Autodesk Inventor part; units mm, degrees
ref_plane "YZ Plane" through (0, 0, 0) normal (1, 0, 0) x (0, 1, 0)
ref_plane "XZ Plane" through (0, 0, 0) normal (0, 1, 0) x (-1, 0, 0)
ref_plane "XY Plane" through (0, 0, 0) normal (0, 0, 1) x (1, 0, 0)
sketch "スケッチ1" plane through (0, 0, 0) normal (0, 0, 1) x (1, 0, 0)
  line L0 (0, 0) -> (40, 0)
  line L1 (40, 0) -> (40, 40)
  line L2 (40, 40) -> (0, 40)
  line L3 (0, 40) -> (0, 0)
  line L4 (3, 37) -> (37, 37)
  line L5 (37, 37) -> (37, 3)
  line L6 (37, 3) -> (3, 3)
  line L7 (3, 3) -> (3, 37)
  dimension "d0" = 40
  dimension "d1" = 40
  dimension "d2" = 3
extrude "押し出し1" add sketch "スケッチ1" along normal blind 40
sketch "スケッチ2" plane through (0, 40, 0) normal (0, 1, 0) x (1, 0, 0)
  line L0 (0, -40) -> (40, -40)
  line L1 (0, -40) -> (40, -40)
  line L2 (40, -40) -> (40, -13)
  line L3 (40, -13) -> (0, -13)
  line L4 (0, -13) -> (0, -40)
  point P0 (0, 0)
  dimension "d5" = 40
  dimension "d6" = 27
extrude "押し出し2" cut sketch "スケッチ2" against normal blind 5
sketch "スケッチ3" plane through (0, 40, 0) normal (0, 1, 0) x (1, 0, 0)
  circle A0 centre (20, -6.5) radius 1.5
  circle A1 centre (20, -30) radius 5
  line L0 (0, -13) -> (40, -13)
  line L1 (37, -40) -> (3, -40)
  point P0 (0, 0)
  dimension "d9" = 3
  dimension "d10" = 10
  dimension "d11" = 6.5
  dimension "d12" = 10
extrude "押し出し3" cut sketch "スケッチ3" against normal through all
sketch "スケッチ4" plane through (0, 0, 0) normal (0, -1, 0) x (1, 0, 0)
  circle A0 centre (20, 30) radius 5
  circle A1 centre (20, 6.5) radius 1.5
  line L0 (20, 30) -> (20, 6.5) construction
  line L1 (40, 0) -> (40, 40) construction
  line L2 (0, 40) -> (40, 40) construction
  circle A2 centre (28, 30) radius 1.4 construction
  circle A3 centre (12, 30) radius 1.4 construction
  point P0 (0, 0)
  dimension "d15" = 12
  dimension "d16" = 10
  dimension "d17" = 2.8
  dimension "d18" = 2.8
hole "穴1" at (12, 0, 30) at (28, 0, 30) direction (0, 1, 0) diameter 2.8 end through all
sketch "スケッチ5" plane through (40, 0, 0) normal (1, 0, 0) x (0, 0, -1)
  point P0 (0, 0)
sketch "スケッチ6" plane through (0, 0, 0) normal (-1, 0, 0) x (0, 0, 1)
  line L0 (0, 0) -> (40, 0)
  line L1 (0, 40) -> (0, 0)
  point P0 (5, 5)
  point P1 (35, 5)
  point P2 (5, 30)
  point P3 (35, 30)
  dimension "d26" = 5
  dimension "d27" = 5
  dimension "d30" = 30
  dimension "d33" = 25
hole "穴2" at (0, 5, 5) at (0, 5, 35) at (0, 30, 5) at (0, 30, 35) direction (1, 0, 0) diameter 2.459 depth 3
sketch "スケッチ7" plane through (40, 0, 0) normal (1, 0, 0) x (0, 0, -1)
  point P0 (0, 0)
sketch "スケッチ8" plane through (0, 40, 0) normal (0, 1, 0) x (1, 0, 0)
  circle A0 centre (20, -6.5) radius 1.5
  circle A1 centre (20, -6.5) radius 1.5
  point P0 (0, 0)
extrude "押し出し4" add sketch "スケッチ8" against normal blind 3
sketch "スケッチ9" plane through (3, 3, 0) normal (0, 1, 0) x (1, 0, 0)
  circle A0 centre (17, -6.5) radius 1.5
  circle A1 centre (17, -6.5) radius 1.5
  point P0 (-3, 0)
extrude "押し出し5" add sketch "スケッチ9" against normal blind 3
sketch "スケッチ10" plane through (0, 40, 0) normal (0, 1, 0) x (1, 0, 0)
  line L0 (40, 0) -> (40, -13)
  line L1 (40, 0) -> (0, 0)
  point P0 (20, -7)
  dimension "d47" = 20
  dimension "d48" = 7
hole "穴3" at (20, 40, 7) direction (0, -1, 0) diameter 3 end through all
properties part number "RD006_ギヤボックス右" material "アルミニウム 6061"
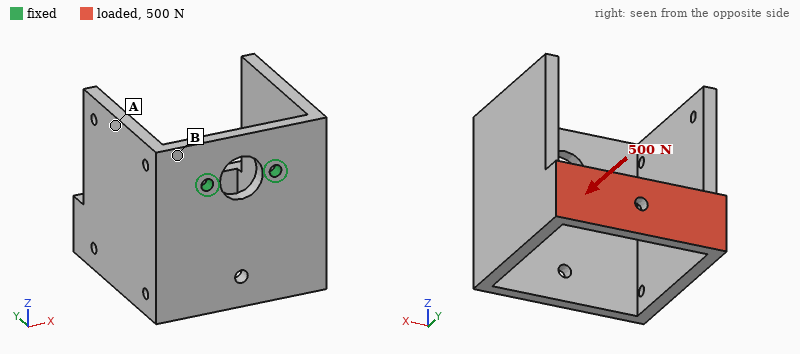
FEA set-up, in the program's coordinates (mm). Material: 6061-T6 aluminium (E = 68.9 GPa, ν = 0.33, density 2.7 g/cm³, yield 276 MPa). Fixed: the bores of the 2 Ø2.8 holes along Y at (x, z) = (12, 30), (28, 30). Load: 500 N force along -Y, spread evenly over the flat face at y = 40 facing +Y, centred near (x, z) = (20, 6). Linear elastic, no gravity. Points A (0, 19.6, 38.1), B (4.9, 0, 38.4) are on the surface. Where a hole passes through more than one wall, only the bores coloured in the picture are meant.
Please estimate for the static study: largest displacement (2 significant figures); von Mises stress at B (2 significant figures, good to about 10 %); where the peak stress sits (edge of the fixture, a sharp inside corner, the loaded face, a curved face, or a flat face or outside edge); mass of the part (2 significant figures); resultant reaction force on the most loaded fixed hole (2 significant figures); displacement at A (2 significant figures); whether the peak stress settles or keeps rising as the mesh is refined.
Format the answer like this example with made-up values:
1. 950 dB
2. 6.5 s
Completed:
1. 0.57 mm
2. 58 MPa
3. edge of the fixture
4. 37 g
5. 250 N
6. 0.20 mm
7. keeps rising
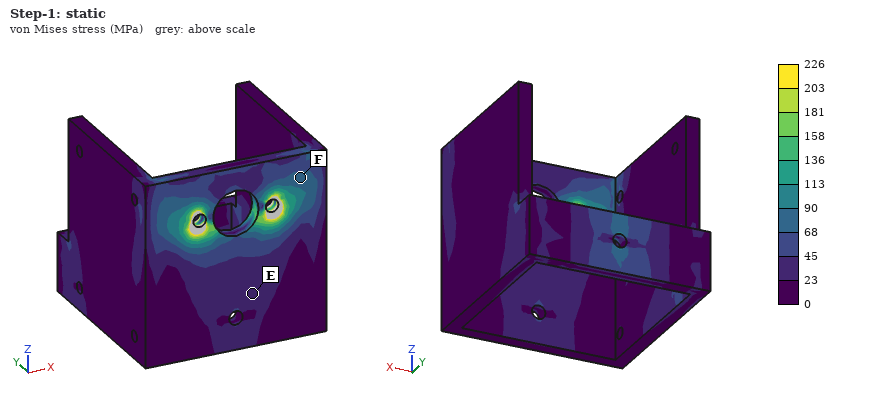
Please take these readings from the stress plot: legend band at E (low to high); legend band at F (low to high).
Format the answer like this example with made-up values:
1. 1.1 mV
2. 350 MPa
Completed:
1. 23 to 45 MPa
2. 68 to 90 MPa
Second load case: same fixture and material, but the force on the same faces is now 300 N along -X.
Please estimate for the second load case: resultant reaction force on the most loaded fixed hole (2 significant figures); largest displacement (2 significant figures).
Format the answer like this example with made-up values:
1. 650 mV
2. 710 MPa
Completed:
1. 550 N
2. 0.58 mm
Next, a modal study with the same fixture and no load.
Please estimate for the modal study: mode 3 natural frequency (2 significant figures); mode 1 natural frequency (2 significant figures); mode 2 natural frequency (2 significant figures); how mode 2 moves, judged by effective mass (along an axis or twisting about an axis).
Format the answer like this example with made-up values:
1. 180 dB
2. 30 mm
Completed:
1. 2500 Hz
2. 1100 Hz
3. 1100 Hz
4. along X
